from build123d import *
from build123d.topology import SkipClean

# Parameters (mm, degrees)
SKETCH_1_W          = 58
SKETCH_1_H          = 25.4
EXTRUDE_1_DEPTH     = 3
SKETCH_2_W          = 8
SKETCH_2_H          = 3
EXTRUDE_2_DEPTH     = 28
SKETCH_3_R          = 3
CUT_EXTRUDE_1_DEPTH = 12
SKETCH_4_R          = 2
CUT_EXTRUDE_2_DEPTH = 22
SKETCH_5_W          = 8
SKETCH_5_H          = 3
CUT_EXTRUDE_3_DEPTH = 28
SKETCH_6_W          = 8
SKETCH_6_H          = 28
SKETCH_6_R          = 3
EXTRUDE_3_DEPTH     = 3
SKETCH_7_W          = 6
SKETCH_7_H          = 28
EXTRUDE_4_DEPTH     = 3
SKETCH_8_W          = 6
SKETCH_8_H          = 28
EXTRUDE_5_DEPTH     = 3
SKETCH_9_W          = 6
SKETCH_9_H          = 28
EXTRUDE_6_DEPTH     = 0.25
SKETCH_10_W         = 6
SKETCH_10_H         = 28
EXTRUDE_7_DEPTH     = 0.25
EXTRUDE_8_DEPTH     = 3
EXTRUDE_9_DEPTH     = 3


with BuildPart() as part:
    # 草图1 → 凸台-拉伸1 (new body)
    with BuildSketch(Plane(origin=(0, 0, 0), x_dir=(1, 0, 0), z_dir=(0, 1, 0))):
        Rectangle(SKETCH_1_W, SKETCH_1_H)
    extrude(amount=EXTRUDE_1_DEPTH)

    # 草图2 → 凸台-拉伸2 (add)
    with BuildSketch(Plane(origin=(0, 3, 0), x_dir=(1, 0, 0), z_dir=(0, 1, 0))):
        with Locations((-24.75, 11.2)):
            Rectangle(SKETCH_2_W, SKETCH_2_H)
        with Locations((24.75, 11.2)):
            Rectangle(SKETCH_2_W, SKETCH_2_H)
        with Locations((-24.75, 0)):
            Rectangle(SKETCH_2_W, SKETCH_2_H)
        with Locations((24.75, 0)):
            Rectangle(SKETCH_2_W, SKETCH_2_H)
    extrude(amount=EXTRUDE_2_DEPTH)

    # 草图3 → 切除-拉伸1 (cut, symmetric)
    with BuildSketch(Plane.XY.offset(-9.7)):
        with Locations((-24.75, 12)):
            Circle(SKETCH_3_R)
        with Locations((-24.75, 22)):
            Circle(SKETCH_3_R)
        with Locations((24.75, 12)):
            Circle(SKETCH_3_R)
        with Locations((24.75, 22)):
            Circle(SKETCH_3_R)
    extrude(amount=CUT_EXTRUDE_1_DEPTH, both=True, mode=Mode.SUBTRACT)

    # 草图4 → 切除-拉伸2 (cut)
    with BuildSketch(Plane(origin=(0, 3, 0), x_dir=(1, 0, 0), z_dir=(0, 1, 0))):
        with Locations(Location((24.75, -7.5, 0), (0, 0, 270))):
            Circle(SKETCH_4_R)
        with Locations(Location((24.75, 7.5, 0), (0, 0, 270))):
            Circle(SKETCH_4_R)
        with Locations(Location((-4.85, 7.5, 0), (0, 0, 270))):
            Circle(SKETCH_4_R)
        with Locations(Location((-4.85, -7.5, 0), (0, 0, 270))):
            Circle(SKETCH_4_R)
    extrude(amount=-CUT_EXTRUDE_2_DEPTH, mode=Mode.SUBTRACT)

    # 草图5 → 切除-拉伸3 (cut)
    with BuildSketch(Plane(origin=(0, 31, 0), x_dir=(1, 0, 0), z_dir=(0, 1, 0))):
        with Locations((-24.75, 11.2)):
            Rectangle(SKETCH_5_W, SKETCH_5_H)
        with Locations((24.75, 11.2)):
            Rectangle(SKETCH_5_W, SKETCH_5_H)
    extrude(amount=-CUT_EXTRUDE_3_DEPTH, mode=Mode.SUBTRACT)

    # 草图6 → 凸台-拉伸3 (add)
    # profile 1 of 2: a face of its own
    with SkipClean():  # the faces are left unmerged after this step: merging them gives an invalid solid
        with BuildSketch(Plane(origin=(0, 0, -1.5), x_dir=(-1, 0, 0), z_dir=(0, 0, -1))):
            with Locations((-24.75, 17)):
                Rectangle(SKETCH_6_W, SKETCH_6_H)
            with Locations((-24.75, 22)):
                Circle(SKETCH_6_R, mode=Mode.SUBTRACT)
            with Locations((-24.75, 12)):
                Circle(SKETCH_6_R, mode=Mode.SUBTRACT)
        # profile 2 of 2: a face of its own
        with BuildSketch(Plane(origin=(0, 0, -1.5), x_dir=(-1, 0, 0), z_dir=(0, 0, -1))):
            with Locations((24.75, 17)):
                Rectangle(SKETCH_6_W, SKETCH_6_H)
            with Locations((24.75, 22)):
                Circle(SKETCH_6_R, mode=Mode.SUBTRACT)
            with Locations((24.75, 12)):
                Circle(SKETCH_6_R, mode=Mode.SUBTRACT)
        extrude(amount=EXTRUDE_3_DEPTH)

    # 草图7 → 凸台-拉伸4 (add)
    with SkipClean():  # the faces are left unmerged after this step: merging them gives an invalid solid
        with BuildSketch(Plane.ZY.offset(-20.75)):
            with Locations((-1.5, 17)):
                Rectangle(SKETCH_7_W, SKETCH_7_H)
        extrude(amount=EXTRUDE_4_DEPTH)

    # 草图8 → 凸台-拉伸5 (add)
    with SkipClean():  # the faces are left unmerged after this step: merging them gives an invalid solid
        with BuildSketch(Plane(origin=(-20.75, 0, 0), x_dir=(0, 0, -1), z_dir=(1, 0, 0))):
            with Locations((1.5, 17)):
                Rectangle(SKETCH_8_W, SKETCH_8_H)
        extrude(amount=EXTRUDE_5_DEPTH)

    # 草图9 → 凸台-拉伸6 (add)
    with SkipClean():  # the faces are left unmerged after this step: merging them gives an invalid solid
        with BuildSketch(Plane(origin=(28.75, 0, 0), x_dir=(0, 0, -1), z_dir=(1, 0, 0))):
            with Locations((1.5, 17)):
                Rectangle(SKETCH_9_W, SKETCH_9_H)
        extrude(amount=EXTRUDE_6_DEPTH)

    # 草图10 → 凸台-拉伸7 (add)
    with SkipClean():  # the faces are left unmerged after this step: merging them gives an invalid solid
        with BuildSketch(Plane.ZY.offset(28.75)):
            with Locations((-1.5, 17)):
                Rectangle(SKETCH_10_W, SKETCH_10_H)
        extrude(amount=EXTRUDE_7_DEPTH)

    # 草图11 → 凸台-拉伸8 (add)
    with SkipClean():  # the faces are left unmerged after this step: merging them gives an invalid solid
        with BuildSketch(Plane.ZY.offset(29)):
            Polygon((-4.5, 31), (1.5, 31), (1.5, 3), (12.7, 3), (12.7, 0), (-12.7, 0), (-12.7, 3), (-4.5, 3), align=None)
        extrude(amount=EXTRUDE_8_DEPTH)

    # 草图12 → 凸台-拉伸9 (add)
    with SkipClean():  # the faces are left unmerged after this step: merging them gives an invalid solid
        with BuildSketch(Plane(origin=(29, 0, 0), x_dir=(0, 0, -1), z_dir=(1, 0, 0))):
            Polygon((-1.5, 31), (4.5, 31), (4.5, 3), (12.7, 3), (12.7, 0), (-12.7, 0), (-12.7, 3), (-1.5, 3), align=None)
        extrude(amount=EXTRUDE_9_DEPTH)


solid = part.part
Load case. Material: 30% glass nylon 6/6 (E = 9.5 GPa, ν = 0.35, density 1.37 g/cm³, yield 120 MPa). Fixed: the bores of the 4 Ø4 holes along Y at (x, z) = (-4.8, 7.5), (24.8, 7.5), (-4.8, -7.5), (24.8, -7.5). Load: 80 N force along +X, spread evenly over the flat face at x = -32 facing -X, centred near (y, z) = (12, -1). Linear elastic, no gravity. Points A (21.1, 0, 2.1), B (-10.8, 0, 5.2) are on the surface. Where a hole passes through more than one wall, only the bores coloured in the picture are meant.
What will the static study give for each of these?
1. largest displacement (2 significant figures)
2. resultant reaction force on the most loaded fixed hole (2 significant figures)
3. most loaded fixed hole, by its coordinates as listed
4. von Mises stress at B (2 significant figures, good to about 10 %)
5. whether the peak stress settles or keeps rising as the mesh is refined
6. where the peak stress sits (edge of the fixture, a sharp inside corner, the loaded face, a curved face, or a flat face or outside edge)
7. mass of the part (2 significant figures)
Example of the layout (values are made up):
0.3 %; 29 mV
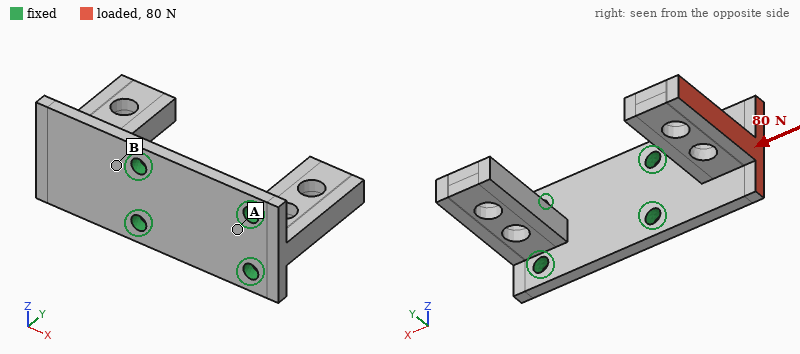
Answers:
0.81 mm; 44 N; (-4.8, -7.5); 19 MPa; keeps rising; edge of the fixture; 12 g
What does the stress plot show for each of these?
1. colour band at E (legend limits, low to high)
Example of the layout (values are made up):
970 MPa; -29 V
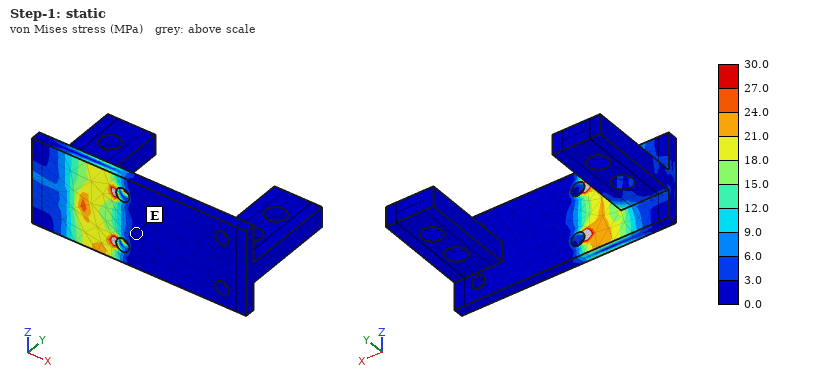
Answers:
0.0 to 3.0 MPa
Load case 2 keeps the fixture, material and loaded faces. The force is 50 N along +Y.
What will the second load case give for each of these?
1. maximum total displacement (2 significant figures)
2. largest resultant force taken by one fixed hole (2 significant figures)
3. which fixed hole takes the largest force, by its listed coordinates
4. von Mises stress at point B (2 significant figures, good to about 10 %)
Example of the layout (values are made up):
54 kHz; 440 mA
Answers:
0.90 mm; 29 N; (-4.8, -7.5); 25 MPa
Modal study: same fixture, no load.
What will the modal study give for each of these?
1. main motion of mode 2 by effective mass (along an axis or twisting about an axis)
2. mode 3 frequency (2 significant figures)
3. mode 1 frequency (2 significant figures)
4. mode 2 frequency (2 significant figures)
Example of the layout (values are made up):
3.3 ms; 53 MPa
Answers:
along Z; 2400 Hz; 770 Hz; 1300 Hz
